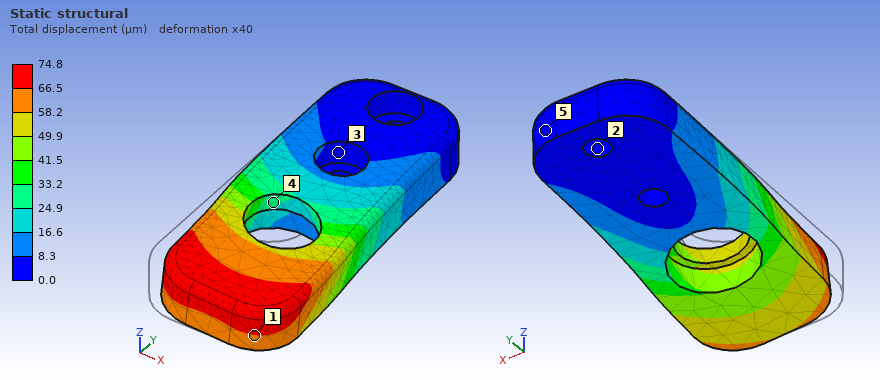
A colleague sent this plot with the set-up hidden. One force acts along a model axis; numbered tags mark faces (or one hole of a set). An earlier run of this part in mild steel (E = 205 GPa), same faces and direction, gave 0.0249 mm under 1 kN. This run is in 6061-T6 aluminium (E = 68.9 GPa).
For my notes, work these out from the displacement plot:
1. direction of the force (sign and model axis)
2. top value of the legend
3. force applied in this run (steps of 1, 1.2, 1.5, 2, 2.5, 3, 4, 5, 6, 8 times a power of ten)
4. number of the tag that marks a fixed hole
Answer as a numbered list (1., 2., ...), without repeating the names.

1. +X
2. 74.8 µm
3. 1 kN
4. 2
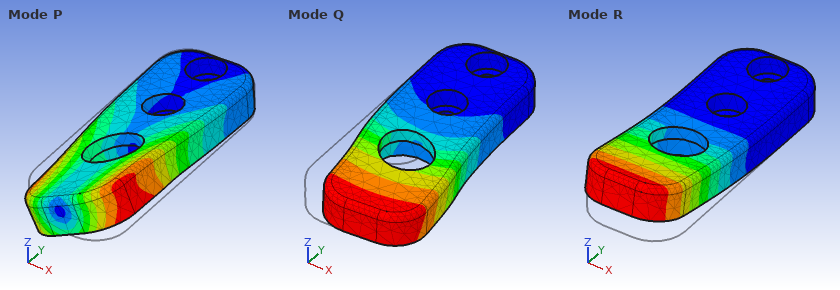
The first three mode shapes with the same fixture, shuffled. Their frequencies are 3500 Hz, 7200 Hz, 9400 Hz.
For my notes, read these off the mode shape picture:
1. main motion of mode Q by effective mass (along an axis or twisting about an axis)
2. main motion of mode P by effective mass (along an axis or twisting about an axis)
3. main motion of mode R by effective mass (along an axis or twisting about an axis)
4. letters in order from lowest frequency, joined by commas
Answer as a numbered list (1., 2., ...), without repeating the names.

1. along X
2. twisting about Y
3. along Z
4. R, Q, P
